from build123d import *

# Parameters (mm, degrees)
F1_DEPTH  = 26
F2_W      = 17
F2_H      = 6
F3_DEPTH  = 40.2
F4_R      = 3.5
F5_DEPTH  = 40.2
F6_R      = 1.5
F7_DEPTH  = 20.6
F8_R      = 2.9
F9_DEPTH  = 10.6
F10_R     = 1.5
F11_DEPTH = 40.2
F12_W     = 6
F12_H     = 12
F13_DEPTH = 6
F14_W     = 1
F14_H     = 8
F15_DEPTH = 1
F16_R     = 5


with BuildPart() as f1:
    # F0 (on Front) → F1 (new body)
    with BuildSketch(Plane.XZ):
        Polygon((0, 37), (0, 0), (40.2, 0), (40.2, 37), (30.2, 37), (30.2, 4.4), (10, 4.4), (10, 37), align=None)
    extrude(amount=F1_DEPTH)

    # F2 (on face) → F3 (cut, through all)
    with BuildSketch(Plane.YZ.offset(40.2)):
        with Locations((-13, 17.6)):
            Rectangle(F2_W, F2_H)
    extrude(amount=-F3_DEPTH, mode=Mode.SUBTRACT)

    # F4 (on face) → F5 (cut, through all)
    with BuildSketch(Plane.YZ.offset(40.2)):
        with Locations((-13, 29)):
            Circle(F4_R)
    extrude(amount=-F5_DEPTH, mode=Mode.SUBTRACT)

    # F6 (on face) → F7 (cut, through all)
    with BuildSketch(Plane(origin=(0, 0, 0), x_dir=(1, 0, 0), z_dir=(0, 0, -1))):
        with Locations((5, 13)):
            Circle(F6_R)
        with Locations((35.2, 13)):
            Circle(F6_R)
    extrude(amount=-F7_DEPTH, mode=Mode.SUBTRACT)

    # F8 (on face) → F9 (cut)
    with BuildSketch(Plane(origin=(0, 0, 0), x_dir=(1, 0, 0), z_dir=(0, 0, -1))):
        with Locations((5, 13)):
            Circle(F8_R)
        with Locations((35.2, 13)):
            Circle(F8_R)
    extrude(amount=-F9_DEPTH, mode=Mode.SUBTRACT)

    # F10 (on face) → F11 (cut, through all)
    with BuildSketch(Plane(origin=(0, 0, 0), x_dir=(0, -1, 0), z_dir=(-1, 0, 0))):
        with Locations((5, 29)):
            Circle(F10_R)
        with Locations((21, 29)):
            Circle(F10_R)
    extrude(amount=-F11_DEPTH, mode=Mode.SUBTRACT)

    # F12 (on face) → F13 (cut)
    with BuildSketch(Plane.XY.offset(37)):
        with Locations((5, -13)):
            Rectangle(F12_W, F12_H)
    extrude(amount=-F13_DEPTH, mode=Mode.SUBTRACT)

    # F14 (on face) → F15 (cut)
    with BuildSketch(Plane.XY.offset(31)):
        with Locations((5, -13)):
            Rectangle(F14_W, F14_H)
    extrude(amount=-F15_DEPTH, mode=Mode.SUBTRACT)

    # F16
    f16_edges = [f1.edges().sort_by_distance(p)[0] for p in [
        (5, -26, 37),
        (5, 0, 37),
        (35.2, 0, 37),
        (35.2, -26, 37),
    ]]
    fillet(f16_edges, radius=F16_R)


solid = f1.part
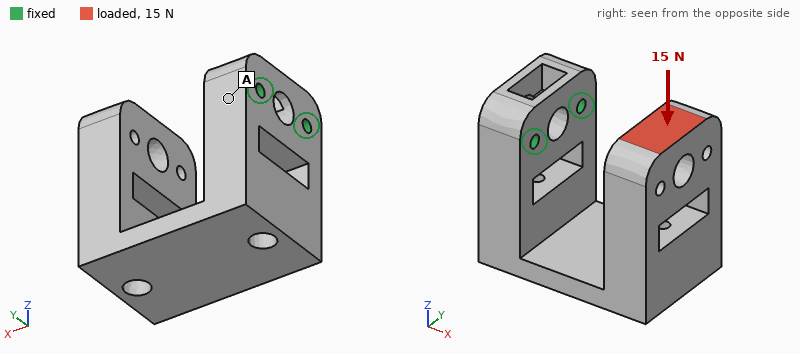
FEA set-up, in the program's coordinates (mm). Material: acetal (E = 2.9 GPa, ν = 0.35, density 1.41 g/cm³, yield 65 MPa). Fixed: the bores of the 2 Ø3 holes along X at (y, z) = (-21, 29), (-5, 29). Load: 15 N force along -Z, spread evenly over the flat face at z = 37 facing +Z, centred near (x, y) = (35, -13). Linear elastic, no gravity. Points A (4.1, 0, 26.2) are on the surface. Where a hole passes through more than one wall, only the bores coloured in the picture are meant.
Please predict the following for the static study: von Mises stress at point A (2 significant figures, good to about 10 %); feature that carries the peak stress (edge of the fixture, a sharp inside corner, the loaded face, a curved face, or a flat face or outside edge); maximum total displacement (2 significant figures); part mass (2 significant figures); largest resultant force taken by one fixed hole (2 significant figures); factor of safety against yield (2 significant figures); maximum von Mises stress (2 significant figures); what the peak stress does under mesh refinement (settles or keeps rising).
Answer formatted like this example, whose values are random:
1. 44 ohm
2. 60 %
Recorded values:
1. 0.71 MPa
2. a flat face or outside edge
3. 0.58 mm
4. 24 g
5. 7.6 N
6. 15
7. 4.3 MPa
8. settles
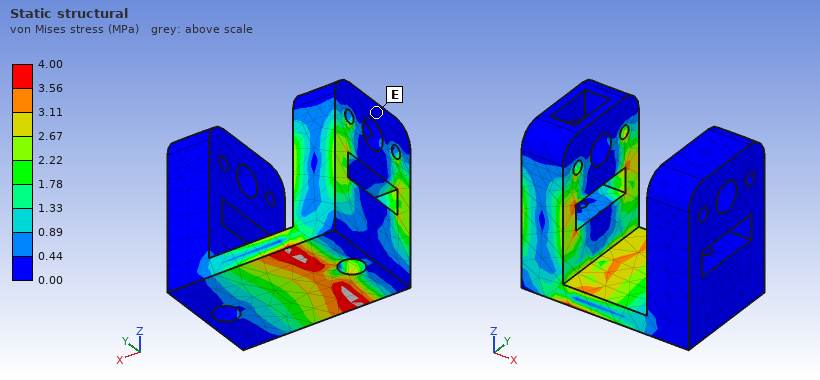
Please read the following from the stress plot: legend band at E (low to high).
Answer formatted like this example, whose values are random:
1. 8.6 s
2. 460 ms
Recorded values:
1. 0.00 to 0.44 MPa
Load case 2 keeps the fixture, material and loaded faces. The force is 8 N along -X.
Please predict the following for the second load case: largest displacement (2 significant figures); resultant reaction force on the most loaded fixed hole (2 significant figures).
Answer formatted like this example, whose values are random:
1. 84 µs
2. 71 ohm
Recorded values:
1. 0.58 mm
2. 4.0 N
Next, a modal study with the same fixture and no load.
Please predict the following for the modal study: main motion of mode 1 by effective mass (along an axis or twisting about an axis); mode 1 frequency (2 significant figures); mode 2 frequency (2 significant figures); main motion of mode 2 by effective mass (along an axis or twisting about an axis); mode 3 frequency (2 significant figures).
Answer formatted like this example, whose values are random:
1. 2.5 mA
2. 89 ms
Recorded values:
1. along Z
2. 250 Hz
3. 390 Hz
4. along Y
5. 620 Hz
